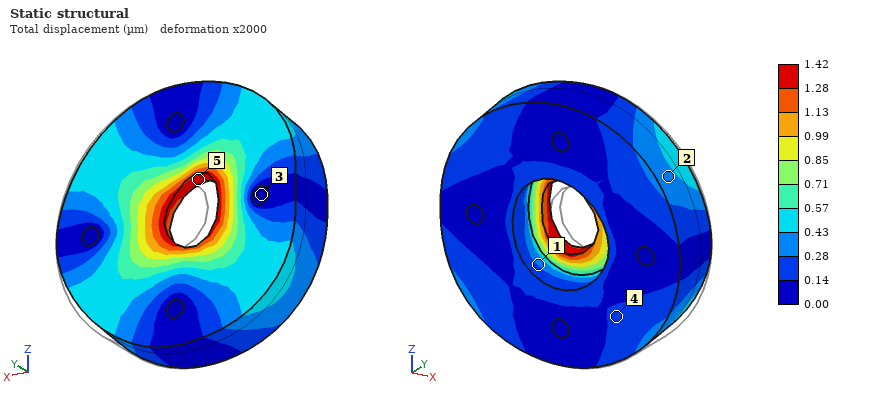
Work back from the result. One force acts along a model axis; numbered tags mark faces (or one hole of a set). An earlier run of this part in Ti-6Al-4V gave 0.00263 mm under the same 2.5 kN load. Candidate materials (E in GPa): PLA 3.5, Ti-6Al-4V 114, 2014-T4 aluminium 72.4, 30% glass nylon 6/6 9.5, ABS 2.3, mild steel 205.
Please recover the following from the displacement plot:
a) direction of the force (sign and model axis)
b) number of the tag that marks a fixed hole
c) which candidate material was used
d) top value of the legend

-X
3
mild steel
1.42 µm
